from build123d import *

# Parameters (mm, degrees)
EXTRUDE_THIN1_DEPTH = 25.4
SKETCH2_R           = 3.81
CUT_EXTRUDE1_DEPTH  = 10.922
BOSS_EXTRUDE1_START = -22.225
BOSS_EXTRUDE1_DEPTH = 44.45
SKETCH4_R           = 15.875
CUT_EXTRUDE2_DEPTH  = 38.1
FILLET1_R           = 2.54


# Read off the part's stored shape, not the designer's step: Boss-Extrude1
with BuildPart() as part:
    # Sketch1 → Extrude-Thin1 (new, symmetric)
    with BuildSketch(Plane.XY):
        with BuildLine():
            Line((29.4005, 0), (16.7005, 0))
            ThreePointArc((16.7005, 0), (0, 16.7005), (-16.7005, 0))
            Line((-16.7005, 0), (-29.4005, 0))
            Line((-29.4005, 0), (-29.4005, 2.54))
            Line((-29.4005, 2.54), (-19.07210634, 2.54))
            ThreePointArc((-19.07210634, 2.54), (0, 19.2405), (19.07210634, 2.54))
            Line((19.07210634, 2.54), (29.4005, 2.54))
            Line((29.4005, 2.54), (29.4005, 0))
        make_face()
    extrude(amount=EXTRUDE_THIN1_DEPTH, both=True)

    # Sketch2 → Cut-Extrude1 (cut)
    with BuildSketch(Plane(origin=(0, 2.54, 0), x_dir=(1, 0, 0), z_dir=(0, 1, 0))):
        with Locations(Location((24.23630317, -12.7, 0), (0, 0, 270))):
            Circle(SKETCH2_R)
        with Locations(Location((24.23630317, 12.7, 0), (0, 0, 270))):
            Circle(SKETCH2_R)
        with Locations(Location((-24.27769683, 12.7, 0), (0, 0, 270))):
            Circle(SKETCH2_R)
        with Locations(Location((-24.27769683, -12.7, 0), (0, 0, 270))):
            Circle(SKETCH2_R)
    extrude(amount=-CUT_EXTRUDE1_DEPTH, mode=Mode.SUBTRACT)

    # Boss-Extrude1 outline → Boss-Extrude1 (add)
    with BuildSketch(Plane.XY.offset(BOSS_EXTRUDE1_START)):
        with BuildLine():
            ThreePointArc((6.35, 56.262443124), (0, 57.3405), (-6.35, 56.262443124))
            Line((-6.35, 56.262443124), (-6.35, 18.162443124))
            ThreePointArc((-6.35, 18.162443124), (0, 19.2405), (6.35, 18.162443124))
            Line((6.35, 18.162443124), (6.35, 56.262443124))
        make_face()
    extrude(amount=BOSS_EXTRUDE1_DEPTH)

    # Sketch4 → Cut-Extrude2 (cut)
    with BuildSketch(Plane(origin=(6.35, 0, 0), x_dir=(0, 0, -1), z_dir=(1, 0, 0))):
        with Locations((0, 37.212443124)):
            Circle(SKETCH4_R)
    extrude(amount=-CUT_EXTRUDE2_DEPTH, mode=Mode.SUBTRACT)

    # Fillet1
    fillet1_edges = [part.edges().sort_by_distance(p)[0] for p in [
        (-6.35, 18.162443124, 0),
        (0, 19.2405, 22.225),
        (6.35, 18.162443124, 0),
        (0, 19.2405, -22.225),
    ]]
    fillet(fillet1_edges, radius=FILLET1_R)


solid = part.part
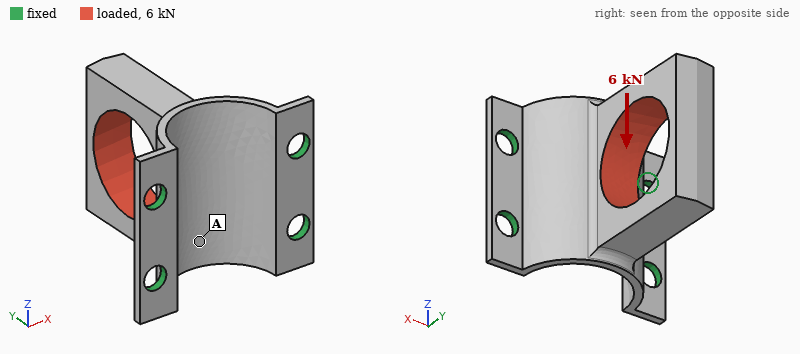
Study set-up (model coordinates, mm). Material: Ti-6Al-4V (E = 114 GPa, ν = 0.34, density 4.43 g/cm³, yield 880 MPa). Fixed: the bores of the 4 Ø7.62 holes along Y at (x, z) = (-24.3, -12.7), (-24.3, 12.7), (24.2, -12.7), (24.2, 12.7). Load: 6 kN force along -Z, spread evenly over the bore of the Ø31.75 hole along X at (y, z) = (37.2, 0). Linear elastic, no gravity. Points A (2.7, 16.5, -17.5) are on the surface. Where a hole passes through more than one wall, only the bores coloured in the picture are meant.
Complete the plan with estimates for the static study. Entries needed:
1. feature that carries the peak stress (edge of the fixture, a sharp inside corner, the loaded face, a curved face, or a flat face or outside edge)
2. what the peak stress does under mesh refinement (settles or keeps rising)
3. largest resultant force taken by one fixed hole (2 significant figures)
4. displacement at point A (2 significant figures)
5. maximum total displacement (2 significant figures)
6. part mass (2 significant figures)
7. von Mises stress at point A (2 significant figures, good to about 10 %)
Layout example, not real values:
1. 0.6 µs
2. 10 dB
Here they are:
1. edge of the fixture
2. keeps rising
3. 4.9 kN
4. 0.081 mm
5. 0.31 mm
6. 93 g
7. 66 MPa
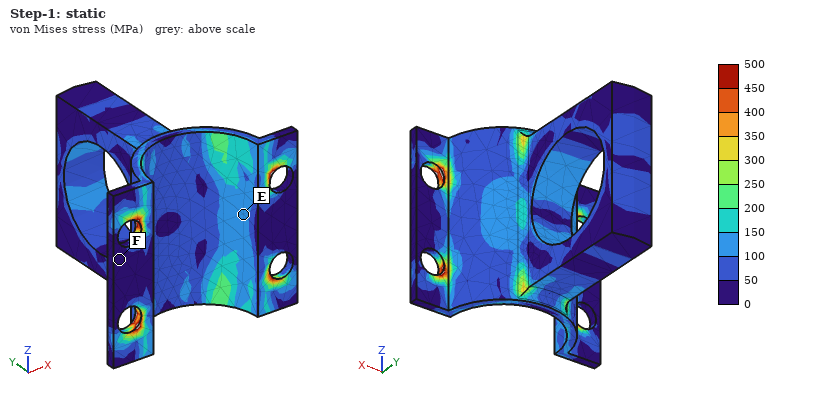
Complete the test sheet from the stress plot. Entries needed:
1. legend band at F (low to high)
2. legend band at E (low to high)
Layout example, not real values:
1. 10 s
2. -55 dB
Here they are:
1. 0 to 50 MPa
2. 100 to 150 MPa
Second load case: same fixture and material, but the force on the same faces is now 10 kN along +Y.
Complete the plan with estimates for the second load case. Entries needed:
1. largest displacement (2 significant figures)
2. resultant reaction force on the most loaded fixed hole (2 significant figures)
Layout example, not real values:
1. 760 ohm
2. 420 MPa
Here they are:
1. 88 µm
2. 3.2 kN
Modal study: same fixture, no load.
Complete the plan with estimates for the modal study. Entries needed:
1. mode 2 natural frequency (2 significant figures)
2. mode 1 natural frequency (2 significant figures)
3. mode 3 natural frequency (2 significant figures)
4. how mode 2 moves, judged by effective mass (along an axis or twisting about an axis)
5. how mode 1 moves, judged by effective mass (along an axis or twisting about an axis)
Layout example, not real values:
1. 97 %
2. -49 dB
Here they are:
1. 3300 Hz
2. 2600 Hz
3. 6300 Hz
4. along Z
5. along X
